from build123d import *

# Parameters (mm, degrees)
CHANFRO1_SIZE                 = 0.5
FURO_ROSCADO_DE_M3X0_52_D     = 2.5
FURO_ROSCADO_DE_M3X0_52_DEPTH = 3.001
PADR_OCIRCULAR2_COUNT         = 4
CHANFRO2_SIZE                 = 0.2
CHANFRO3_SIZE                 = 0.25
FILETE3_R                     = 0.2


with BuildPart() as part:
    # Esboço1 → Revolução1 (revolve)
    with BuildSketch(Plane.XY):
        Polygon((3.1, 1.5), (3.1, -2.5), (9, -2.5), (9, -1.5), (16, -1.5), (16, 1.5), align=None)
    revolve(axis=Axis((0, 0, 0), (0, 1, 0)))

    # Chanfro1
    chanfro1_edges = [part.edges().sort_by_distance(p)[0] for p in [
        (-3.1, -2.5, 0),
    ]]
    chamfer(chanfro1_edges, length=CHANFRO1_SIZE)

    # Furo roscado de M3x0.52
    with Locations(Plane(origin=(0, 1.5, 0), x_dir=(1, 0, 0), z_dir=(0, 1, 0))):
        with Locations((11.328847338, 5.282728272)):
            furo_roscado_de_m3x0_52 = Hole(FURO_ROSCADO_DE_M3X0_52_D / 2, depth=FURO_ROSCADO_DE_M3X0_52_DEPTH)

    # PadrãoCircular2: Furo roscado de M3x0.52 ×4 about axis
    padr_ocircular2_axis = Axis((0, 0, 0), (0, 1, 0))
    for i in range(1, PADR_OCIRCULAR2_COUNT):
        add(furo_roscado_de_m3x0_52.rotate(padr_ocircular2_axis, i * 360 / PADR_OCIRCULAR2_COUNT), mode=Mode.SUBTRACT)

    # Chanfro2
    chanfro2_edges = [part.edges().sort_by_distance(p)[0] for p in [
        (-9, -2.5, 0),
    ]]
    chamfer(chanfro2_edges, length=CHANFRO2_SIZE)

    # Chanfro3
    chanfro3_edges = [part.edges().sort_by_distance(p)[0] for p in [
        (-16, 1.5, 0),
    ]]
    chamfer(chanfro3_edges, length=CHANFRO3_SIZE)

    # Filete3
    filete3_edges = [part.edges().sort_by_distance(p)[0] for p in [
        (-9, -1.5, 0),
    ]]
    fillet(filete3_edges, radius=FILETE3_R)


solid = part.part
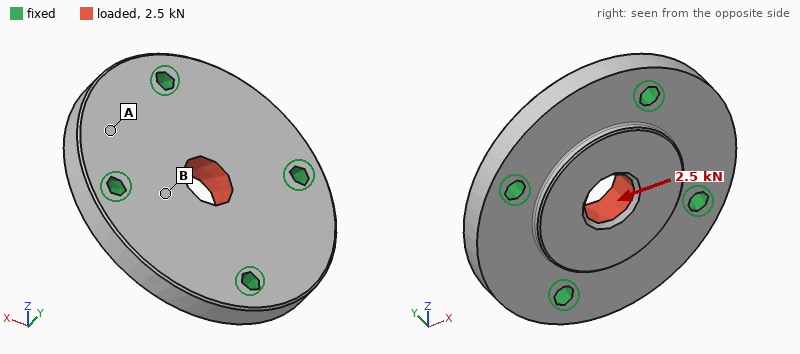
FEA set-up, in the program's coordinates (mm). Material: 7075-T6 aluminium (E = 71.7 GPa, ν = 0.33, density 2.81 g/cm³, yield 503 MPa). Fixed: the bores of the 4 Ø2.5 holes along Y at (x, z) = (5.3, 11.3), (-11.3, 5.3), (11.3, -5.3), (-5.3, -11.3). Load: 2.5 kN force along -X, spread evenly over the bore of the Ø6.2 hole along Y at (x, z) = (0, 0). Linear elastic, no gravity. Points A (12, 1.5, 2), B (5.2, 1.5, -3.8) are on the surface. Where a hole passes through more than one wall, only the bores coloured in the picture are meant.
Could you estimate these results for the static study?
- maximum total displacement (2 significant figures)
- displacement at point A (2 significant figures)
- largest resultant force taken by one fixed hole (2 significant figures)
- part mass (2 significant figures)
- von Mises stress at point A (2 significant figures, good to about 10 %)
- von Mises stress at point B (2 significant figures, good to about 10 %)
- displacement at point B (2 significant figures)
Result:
5.4 µm
2.7 µm
760 N
7.0 g
9.6 MPa
37 MPa
2.8 µm
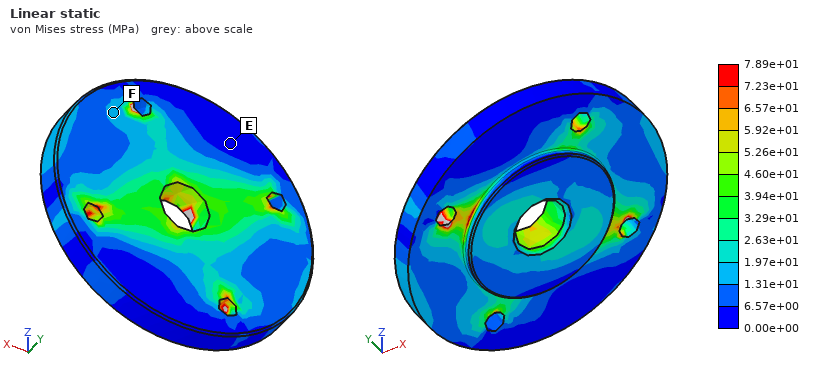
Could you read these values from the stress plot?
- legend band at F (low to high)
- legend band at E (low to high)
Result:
1.31e+01 to 1.97e+01 MPa
0.00e+00 to 6.57e+00 MPa
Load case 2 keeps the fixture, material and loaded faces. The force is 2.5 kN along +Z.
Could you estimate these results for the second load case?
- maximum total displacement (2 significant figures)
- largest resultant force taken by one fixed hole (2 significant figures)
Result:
5.3 µm
760 N
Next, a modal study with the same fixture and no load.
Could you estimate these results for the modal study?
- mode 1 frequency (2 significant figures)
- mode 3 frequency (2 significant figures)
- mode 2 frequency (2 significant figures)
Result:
35 kHz
36 kHz
36 kHz
